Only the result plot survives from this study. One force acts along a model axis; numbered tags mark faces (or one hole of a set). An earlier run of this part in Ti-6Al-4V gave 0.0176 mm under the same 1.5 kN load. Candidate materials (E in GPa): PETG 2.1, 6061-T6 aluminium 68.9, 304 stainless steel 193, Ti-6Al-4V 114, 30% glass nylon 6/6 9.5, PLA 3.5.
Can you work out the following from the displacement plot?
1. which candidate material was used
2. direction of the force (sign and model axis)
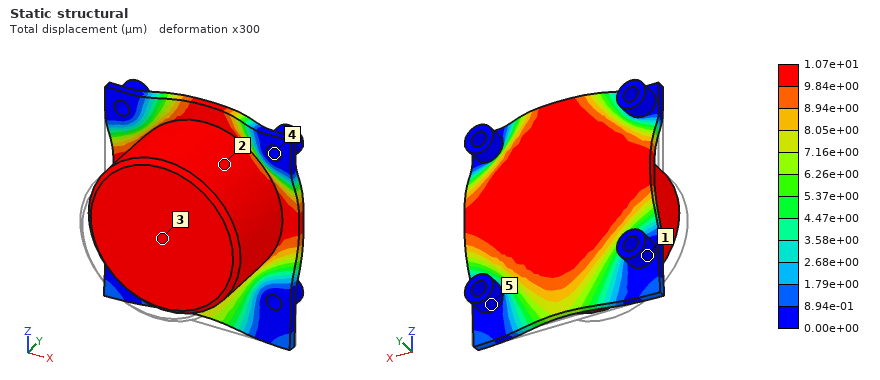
304 stainless steel
+Y
